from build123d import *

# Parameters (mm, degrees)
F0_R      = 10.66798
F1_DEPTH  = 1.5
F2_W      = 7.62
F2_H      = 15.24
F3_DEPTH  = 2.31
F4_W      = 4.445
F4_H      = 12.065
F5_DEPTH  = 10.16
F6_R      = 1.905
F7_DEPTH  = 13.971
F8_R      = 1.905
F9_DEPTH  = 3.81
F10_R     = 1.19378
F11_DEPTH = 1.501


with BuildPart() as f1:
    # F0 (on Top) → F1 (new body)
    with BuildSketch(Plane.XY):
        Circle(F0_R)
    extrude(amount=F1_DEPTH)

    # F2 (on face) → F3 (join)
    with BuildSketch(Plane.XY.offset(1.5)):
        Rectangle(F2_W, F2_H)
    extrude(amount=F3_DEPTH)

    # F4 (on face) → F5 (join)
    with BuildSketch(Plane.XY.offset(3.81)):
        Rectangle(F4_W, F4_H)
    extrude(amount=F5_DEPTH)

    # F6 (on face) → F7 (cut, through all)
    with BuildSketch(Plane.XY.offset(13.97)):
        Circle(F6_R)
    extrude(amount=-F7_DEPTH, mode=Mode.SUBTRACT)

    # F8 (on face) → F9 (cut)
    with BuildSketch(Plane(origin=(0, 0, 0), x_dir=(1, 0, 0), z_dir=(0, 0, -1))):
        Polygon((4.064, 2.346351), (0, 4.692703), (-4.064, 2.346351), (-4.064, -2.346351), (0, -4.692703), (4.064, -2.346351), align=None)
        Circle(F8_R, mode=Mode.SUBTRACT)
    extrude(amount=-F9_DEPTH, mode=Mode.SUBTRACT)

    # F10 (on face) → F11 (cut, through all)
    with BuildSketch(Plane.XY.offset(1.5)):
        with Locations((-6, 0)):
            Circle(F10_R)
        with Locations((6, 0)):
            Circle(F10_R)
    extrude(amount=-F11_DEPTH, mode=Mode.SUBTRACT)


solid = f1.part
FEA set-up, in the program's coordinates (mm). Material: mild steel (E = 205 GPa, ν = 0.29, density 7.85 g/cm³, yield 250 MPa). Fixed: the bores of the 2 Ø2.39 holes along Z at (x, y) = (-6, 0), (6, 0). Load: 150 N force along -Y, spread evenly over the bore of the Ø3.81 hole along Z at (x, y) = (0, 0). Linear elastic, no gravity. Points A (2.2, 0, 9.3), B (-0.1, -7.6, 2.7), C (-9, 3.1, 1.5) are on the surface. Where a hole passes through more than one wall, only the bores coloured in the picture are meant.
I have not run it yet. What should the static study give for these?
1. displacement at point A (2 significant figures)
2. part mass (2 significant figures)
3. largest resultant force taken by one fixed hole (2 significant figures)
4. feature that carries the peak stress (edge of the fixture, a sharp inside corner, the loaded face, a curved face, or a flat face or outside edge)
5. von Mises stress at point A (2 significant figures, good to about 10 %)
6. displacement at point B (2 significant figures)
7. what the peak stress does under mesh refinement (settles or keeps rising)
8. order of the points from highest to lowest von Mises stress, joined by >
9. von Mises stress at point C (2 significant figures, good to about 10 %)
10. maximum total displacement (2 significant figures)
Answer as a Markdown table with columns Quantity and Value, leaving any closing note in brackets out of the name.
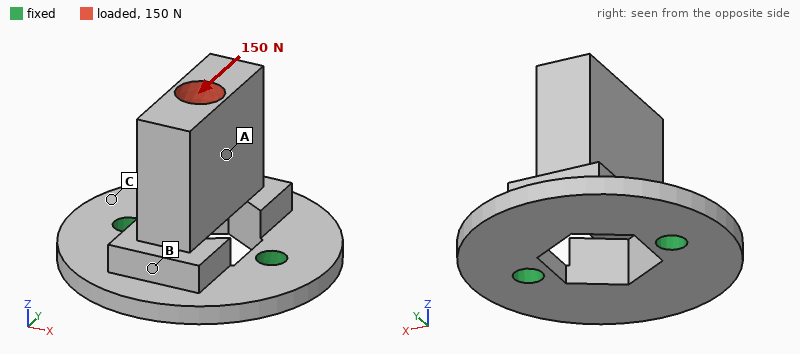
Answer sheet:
| Quantity | Value |
|---|---|
| displacement at point A | 14 µm |
| part mass | 7.9 g |
| largest resultant force taken by one fixed hole | 75 N |
| feature that carries the peak stress | edge of the fixture |
| von Mises stress at point A | 34 MPa |
| displacement at point B | 12 µm |
| what the peak stress does under mesh refinement | keeps rising |
| order of the points from highest to lowest von Mises stress, joined by > | C > A > B |
| von Mises stress at point C | 47 MPa |
| maximum total displacement | 22 µm |
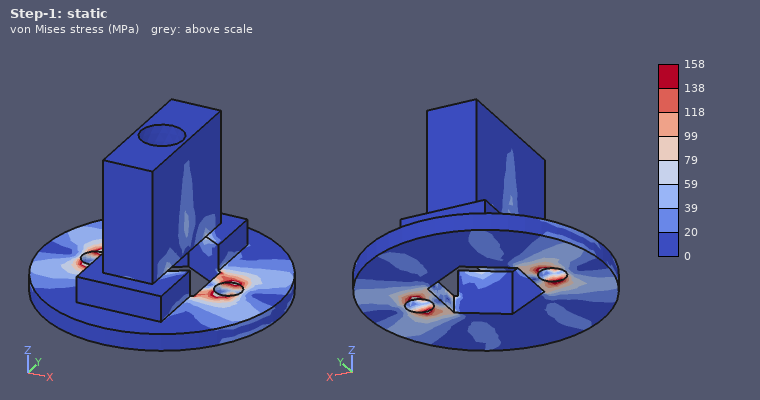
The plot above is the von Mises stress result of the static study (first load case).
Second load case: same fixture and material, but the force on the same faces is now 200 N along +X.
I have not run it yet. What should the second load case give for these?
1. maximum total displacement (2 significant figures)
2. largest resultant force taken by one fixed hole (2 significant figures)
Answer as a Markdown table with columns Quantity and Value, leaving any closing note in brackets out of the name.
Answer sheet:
| Quantity | Value |
|---|---|
| maximum total displacement | 14 µm |
| largest resultant force taken by one fixed hole | 180 N |
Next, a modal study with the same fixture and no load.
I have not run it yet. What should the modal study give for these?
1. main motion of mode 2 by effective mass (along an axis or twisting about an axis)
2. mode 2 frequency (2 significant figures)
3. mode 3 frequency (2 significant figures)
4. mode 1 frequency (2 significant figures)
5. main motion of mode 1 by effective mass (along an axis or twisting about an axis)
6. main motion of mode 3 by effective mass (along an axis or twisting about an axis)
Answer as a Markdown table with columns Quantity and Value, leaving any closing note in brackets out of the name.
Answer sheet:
| Quantity | Value |
|---|---|
| main motion of mode 2 by effective mass | along X |
| mode 2 frequency | 12 kHz |
| mode 3 frequency | 17 kHz |
| mode 1 frequency | 6800 Hz |
| main motion of mode 1 by effective mass | along Y |
| main motion of mode 3 by effective mass | along Z |
